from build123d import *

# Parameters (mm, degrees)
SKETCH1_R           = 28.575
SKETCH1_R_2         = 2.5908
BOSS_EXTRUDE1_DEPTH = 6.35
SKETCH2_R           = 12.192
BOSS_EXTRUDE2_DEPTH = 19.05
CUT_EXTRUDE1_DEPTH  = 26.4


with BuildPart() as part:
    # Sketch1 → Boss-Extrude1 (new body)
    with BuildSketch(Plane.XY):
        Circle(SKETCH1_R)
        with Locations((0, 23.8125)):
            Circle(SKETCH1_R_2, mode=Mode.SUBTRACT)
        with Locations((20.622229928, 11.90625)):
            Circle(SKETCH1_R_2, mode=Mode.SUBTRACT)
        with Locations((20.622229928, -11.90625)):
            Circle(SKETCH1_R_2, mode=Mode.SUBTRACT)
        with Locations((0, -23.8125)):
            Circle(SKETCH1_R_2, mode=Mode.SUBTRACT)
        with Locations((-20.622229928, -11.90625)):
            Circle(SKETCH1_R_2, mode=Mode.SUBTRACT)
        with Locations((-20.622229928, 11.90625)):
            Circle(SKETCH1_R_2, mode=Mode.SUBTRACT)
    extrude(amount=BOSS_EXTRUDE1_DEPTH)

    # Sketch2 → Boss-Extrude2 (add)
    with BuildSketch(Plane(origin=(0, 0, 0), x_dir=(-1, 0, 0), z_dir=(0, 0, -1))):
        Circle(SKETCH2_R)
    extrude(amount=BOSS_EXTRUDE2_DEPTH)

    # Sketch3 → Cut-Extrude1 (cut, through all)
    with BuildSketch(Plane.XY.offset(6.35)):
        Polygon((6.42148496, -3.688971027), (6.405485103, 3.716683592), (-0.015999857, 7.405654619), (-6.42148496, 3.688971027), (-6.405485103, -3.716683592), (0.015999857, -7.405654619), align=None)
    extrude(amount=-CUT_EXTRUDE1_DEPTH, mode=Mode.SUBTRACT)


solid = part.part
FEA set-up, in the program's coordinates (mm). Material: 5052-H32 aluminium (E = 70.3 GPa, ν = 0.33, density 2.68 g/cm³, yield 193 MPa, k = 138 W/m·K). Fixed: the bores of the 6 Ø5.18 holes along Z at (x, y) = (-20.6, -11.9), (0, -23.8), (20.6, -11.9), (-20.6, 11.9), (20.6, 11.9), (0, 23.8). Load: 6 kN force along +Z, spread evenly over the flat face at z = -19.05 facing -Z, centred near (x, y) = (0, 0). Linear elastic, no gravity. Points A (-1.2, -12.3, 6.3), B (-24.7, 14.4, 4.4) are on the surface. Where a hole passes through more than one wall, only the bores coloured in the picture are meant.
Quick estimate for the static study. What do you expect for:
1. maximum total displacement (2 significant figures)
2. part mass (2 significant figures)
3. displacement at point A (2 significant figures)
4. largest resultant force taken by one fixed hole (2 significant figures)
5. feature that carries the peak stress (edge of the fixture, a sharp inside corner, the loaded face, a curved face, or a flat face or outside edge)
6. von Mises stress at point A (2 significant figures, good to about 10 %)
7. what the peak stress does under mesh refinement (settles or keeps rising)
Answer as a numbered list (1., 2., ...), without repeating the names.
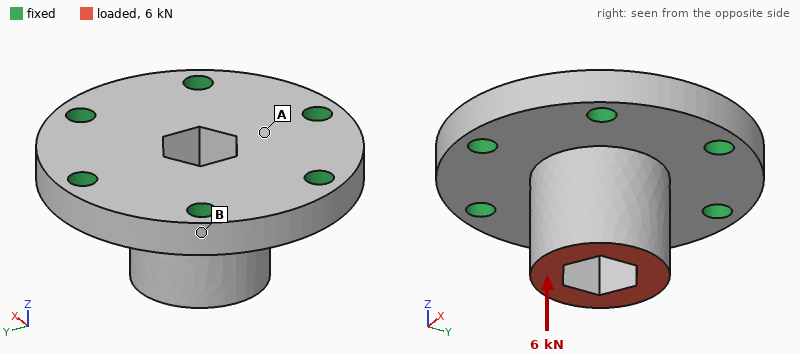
1. 21 µm
2. 56 g
3. 14 µm
4. 1.1 kN
5. edge of the fixture
6. 24 MPa
7. keeps rising
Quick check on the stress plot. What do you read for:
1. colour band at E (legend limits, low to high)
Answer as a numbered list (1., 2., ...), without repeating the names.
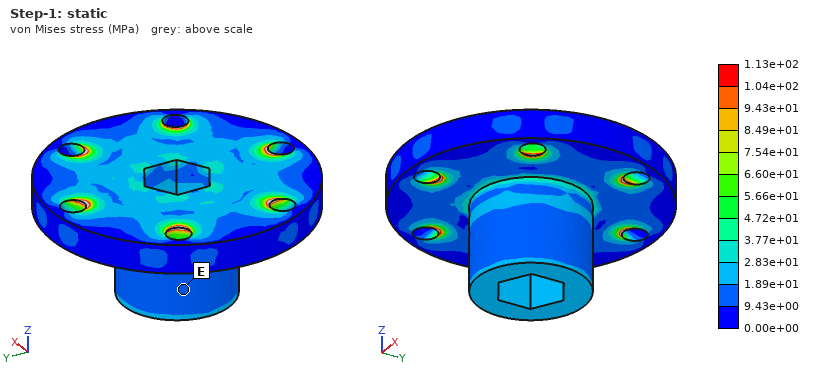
1. 9.43e+00 to 1.89e+01 MPa
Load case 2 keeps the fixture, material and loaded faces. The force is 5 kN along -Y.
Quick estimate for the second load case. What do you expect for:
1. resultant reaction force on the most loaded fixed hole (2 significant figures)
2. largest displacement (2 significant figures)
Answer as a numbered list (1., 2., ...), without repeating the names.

1. 2.4 kN
2. 81 µm
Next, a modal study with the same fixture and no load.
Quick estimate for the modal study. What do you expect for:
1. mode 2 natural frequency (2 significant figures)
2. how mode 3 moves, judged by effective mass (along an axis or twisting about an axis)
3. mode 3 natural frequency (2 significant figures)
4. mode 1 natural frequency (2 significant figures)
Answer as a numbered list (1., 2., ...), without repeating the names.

1. 16 kHz
2. along Z
3. 18 kHz
4. 16 kHz
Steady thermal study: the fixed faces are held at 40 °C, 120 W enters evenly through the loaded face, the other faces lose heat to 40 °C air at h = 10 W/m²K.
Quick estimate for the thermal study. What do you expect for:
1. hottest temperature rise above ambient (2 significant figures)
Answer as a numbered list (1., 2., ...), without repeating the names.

1. 73 K
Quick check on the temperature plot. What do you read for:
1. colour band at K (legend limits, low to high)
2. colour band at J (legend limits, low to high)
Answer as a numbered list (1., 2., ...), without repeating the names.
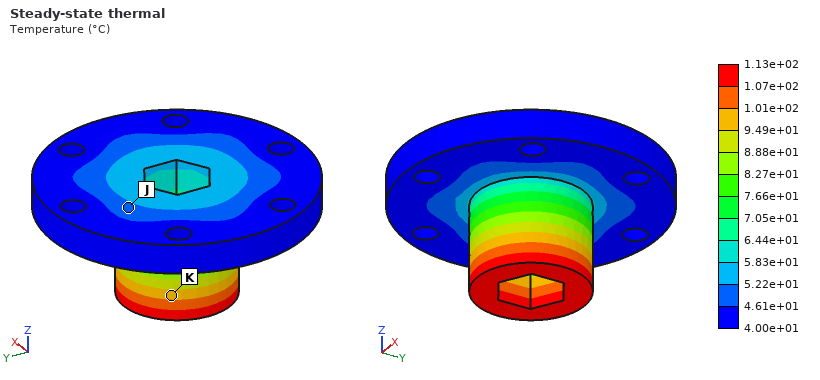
1. 9.49e+01 to 1.01e+02 °C
2. 4.61e+01 to 5.22e+01 °C
